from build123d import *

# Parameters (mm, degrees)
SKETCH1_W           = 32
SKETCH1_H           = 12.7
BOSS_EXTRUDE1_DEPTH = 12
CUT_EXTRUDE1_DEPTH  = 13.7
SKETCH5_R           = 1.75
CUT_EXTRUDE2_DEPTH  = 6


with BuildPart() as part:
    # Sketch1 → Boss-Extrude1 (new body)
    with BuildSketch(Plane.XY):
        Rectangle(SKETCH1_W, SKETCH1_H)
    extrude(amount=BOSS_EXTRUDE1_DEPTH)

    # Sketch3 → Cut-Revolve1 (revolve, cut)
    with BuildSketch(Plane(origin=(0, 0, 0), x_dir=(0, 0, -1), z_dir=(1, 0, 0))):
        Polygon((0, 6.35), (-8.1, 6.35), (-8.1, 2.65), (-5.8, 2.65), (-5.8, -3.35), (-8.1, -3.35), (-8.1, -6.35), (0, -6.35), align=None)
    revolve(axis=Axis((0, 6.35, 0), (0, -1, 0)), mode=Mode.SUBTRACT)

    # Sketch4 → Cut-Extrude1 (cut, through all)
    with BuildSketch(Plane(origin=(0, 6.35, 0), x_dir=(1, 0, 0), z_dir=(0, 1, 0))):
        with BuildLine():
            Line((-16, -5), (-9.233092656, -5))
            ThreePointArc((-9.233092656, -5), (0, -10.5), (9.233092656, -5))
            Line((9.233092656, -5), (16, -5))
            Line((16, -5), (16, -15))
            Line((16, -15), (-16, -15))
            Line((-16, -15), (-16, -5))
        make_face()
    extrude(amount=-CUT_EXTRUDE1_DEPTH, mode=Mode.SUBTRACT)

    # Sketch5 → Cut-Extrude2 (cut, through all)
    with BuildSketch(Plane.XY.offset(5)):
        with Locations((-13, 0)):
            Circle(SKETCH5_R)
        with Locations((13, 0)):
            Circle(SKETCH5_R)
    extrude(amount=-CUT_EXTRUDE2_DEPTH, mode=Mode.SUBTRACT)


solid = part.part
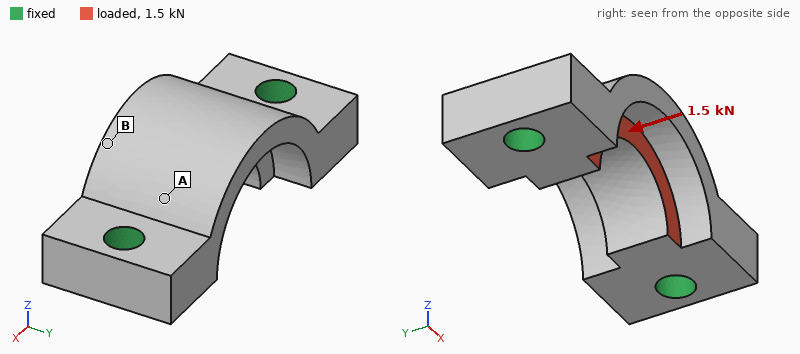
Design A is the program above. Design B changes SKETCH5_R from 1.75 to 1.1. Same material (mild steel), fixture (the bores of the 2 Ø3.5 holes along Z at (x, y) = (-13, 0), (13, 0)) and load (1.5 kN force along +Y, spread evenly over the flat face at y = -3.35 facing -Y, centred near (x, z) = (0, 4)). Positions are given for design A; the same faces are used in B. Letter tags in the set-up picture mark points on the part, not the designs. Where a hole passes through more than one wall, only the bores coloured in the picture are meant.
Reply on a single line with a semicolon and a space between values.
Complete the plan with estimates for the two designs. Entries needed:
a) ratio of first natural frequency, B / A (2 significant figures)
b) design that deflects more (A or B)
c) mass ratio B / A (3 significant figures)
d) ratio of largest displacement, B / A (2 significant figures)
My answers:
0.79; B; 1.03; 1.6
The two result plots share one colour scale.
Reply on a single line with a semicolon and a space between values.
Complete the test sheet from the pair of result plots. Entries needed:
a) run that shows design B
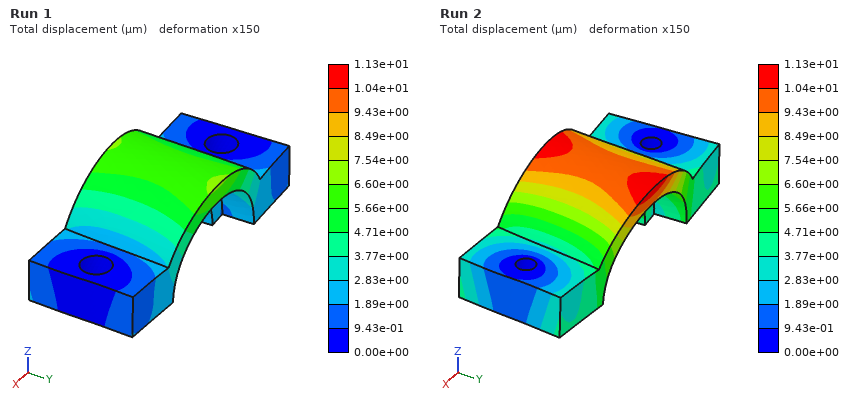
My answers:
Run 2
